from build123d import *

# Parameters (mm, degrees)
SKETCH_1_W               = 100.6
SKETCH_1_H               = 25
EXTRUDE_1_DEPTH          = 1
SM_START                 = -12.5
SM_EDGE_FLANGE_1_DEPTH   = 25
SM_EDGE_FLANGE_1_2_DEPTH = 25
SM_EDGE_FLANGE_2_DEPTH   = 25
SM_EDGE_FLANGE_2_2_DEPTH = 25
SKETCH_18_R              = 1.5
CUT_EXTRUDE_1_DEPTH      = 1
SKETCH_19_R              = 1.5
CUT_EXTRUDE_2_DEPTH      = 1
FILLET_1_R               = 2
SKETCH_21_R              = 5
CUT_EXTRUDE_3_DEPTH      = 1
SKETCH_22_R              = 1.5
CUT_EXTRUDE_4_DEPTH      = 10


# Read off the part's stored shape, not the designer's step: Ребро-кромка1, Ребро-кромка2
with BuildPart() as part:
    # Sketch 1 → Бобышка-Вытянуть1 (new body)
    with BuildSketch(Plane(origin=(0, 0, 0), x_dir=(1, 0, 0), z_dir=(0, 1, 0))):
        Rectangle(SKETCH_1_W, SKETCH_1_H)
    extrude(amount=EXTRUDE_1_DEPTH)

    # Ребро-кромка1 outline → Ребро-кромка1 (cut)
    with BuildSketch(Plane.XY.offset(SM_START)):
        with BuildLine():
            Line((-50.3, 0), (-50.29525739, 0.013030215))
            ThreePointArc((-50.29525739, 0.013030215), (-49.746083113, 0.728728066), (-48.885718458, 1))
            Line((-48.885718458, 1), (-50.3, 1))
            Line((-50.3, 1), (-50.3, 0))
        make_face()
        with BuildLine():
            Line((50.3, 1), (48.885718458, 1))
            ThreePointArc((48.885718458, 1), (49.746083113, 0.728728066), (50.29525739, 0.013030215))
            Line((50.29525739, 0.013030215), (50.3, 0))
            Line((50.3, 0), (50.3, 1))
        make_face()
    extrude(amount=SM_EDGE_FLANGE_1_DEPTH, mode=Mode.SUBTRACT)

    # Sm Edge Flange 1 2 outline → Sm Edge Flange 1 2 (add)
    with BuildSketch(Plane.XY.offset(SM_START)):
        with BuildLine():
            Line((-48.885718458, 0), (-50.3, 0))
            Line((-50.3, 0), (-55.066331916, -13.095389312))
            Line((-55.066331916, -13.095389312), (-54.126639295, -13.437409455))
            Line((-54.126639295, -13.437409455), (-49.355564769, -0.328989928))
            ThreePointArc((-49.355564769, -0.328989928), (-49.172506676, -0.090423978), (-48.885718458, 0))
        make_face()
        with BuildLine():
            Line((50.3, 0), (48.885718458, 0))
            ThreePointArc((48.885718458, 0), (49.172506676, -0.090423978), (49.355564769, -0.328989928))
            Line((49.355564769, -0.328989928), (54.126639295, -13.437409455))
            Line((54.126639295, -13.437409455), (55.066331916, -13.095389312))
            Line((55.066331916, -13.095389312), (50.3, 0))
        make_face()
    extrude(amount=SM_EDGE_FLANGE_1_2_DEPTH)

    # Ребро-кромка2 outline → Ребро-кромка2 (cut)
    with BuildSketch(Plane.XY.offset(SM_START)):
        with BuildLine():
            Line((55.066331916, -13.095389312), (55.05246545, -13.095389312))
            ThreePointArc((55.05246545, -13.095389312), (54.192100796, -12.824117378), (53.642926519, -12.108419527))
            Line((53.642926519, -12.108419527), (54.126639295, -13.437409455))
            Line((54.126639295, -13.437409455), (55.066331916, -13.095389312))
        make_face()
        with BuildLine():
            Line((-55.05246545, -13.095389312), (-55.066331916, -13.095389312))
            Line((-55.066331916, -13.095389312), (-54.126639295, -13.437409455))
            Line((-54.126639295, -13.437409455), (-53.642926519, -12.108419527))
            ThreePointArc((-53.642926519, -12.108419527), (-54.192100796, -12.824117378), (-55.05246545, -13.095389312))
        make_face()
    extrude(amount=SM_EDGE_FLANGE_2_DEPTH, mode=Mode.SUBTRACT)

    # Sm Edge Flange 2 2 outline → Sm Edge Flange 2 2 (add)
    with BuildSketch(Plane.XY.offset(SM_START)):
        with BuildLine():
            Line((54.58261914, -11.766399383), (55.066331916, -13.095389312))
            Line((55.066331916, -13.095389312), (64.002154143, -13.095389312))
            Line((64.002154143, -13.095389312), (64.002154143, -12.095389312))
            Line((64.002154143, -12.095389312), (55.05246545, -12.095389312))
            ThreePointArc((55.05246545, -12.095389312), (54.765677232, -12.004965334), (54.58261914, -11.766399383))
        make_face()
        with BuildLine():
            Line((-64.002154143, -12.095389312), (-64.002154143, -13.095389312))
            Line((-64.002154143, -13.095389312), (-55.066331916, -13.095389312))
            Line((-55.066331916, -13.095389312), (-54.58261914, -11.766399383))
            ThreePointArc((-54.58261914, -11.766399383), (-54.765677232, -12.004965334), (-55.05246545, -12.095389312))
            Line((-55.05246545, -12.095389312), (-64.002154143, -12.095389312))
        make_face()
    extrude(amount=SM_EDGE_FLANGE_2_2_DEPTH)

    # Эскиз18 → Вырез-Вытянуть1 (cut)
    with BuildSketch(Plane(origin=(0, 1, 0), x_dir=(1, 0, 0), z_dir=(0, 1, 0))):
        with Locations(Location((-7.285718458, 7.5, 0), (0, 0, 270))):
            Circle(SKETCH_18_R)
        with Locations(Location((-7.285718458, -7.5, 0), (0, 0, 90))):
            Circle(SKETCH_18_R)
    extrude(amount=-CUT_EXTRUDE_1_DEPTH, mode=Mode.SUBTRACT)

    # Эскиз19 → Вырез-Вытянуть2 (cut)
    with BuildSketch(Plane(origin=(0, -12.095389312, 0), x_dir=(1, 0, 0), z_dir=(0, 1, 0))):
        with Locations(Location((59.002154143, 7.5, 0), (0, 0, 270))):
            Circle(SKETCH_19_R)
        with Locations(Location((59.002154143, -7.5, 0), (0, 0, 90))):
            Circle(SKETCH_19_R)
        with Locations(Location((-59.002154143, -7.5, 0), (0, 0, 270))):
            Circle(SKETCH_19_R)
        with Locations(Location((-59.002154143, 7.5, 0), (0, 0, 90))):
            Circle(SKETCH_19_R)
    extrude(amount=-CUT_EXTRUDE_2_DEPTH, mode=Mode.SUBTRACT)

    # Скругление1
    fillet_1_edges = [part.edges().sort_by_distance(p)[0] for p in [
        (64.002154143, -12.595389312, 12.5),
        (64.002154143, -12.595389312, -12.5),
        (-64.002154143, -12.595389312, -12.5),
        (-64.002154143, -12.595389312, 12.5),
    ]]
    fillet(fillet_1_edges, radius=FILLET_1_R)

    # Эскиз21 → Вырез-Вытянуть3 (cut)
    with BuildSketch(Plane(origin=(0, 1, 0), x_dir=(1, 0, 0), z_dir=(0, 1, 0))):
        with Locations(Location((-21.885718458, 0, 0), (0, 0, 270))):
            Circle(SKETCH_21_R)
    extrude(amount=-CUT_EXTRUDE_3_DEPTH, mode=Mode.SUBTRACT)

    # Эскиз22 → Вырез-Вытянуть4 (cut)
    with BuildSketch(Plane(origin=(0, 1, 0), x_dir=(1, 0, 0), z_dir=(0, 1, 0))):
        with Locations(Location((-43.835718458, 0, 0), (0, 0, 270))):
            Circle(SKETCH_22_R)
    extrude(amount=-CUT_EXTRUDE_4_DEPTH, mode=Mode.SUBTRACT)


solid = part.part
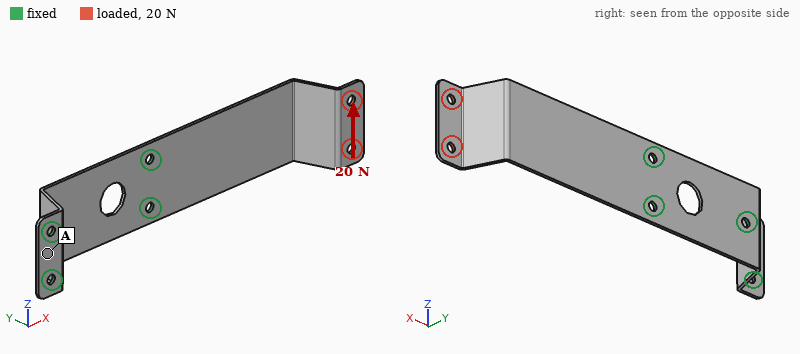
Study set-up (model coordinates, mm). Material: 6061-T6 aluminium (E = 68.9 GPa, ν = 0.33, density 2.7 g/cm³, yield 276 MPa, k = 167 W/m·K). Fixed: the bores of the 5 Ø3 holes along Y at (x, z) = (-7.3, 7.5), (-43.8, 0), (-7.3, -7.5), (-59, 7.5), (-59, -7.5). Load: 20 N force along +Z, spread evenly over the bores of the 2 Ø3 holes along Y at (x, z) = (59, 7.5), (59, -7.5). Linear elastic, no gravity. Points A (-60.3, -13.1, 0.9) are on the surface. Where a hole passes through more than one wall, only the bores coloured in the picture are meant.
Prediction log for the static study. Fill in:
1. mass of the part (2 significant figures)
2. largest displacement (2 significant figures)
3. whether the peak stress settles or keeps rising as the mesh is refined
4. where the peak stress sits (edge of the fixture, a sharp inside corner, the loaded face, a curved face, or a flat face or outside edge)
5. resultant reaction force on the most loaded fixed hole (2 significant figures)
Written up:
9.5 g
1.1 mm
keeps rising
edge of the fixture
76 N
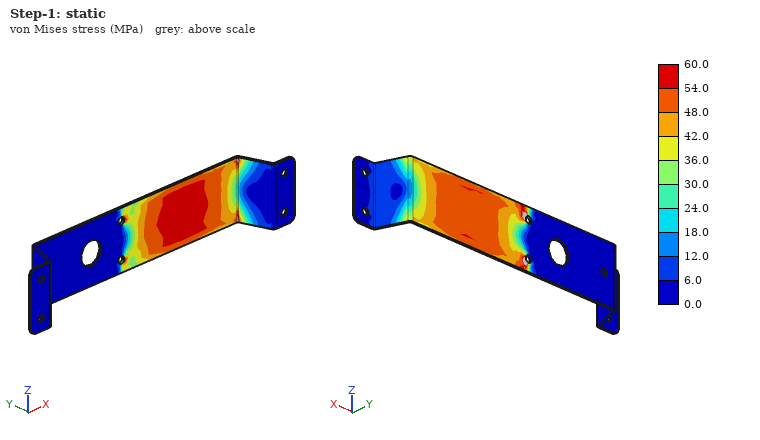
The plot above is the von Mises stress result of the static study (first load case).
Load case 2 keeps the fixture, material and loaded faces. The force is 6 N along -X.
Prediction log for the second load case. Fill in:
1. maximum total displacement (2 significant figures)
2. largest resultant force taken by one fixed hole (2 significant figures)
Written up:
1.4 mm
2.9 N
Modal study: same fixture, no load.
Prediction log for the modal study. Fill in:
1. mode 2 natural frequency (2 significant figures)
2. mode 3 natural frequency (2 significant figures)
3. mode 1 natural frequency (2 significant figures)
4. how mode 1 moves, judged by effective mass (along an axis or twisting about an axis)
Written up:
610 Hz
820 Hz
150 Hz
along Y
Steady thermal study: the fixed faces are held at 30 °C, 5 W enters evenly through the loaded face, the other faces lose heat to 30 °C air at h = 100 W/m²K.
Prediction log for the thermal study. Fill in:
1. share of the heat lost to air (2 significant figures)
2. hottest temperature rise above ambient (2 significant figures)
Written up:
88 %
31 K
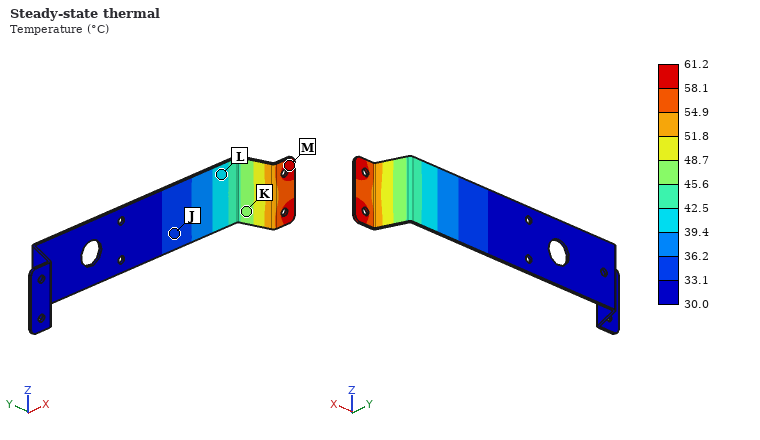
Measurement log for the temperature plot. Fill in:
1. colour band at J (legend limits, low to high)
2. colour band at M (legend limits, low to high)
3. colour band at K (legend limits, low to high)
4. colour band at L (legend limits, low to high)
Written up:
33.1 to 36.2 °C
58.1 to 61.2 °C
45.6 to 48.7 °C
39.4 to 42.5 °C
